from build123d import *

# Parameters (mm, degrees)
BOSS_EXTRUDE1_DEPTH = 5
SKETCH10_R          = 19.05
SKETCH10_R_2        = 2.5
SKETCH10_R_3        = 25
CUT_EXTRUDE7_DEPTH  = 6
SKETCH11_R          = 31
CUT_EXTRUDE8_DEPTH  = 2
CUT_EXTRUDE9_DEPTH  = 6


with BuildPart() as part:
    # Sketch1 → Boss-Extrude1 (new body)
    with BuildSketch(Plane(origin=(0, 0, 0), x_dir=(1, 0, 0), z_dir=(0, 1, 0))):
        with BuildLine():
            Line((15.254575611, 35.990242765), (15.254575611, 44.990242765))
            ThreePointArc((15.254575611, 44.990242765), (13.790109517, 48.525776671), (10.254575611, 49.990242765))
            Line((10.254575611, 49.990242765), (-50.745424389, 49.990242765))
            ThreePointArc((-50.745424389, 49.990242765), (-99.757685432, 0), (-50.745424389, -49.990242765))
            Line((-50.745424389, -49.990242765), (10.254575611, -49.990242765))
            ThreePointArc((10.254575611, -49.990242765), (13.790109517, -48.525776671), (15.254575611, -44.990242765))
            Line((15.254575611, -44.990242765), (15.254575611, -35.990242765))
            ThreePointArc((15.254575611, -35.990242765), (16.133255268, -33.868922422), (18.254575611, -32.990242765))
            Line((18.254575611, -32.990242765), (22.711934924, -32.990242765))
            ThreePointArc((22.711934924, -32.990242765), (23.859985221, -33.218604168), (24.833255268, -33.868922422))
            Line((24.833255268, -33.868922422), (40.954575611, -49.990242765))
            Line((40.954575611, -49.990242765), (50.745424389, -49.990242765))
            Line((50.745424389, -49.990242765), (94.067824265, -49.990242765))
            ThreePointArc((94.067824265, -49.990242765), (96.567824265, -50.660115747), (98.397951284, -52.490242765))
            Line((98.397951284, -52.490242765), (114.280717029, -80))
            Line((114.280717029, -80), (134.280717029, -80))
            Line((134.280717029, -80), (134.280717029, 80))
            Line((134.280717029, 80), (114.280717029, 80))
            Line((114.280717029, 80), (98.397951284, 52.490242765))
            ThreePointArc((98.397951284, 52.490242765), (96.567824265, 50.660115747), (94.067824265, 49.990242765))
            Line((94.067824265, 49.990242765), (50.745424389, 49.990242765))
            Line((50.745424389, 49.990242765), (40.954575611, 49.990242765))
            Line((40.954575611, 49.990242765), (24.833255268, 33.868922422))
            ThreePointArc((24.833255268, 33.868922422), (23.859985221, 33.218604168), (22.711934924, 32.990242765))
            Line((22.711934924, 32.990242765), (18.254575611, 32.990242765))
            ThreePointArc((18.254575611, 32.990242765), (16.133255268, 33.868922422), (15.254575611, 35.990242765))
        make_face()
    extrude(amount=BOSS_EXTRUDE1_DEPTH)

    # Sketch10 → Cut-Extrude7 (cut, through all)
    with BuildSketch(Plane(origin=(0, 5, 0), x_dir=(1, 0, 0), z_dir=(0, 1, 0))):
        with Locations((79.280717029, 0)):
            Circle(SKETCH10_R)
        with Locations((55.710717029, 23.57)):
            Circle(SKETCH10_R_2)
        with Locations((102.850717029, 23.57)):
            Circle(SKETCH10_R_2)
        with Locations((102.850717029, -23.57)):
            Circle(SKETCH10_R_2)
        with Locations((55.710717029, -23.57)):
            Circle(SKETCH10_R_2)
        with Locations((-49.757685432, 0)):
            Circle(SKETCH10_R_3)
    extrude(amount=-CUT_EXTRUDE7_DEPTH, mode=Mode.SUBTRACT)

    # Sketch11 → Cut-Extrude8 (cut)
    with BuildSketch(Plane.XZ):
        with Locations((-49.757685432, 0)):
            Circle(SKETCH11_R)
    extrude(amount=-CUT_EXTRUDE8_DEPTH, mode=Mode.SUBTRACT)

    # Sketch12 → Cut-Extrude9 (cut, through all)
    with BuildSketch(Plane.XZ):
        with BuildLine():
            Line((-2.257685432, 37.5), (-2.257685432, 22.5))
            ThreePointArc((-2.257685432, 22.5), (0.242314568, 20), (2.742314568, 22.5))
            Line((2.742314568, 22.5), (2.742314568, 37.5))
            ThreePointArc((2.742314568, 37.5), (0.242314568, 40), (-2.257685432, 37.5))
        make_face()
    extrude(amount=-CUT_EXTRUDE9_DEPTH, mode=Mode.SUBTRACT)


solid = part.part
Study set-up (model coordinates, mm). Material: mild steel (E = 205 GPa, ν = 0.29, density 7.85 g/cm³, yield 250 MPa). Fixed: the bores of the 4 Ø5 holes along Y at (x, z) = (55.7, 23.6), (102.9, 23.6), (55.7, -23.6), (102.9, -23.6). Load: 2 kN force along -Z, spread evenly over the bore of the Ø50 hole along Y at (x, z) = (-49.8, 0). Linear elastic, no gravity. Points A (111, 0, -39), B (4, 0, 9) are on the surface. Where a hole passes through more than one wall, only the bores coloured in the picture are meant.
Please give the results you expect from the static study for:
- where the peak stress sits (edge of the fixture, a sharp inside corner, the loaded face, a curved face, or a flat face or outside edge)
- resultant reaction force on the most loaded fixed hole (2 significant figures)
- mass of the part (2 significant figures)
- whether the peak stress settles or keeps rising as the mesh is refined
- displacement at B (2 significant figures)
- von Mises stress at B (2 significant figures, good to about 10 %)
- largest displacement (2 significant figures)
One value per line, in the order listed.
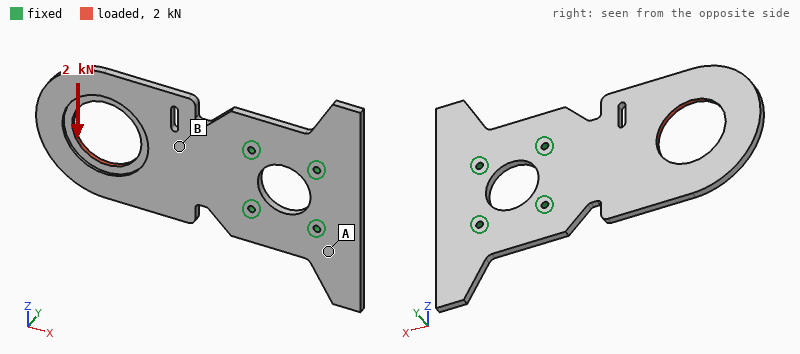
edge of the fixture
3.1 kN
780 g
keeps rising
11 µm
16 MPa
63 µm
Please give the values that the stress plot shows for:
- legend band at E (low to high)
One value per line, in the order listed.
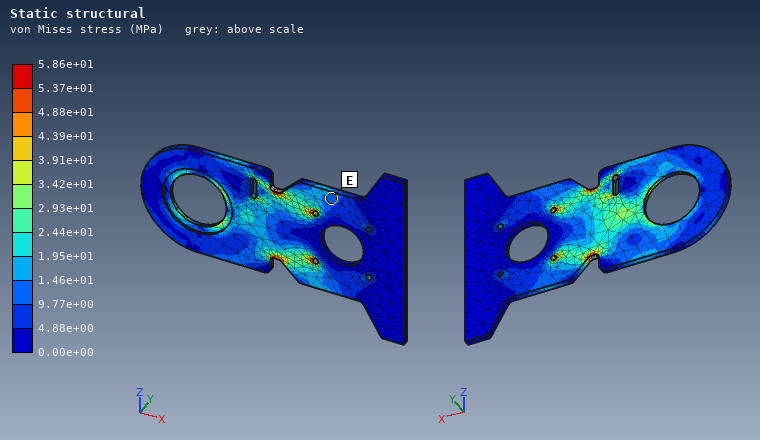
9.77e+00 to 1.46e+01 MPa
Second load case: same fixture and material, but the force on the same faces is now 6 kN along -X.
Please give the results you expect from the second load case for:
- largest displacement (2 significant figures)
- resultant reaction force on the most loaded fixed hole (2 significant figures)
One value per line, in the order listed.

0.40 mm
2.7 kN
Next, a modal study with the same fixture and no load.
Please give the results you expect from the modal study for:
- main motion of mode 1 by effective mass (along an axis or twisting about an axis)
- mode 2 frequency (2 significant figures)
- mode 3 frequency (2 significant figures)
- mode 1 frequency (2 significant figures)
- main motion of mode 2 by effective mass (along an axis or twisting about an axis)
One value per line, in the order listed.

along Y
590 Hz
970 Hz
190 Hz
twisting about X
